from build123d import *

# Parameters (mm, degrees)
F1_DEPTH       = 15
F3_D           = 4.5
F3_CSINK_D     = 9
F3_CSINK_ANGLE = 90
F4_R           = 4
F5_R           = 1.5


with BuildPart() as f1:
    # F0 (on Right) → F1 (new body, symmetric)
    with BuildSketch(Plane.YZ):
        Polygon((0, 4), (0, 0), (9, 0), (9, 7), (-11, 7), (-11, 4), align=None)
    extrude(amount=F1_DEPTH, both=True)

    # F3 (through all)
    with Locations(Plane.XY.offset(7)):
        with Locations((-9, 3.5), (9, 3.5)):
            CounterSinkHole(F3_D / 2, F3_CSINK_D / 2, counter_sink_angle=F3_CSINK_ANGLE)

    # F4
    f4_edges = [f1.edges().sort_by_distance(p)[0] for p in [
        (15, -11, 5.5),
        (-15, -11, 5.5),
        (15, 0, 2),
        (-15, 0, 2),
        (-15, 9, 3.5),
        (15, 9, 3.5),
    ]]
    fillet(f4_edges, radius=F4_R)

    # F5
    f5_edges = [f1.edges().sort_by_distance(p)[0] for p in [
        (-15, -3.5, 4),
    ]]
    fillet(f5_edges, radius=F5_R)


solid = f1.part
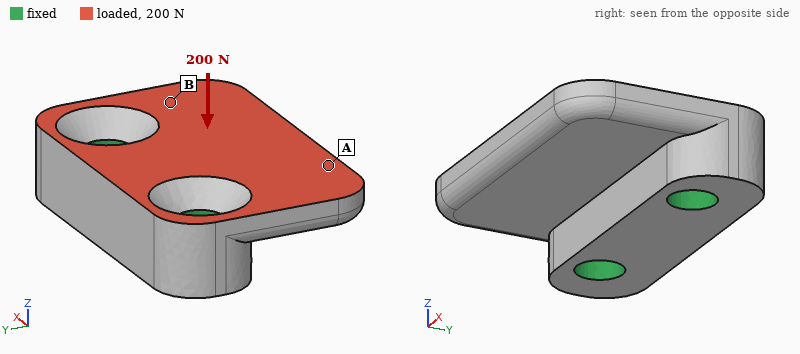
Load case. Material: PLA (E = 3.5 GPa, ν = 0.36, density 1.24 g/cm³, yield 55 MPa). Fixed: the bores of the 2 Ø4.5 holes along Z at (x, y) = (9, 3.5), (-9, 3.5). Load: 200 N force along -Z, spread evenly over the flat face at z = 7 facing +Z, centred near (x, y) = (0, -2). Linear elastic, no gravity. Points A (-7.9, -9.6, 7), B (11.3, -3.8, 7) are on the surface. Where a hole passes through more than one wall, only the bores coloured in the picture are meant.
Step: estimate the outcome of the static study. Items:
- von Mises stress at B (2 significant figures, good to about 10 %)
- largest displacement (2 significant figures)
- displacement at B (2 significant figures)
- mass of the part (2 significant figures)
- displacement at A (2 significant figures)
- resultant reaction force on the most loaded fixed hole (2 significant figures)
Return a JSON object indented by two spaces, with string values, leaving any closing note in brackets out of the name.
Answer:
{
  "von Mises stress at B": "6.2 MPa",
  "largest displacement": "0.25 mm",
  "displacement at B": "0.093 mm",
  "mass of the part": "3.0 g",
  "displacement at A": "0.22 mm",
  "resultant reaction force on the most loaded fixed hole": "100 N"
}
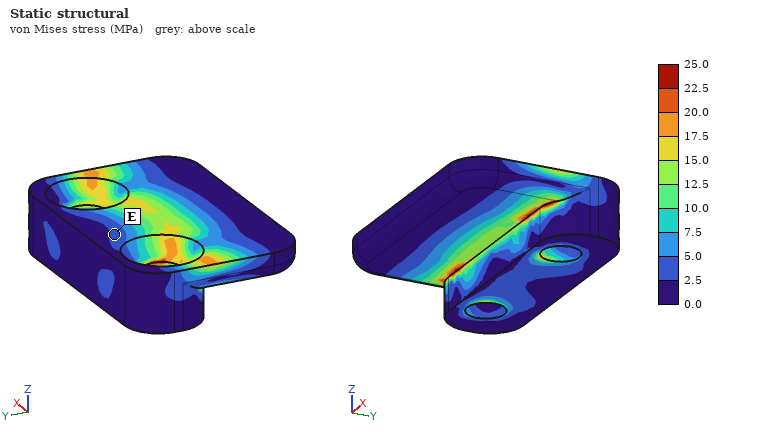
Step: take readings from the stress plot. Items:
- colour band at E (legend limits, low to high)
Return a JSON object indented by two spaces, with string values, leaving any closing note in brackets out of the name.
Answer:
{
  "colour band at E": "2.5 to 5.0 MPa"
}
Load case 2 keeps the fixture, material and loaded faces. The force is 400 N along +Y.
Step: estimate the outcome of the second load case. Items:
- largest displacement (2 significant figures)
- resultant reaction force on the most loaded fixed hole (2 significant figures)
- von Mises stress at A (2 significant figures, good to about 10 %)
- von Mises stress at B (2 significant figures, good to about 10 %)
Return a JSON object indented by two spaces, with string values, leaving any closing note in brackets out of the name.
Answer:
{
  "largest displacement": "0.21 mm",
  "resultant reaction force on the most loaded fixed hole": "200 N",
  "von Mises stress at A": "2.3 MPa",
  "von Mises stress at B": "7.6 MPa"
}
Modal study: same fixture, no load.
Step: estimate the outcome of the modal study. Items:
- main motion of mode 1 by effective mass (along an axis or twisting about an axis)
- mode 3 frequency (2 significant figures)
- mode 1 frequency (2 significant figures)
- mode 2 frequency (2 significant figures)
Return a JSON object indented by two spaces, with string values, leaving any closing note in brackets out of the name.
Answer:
{
  "main motion of mode 1 by effective mass": "along Z",
  "mode 3 frequency": "11 kHz",
  "mode 1 frequency": "4400 Hz",
  "mode 2 frequency": "6300 Hz"
}
